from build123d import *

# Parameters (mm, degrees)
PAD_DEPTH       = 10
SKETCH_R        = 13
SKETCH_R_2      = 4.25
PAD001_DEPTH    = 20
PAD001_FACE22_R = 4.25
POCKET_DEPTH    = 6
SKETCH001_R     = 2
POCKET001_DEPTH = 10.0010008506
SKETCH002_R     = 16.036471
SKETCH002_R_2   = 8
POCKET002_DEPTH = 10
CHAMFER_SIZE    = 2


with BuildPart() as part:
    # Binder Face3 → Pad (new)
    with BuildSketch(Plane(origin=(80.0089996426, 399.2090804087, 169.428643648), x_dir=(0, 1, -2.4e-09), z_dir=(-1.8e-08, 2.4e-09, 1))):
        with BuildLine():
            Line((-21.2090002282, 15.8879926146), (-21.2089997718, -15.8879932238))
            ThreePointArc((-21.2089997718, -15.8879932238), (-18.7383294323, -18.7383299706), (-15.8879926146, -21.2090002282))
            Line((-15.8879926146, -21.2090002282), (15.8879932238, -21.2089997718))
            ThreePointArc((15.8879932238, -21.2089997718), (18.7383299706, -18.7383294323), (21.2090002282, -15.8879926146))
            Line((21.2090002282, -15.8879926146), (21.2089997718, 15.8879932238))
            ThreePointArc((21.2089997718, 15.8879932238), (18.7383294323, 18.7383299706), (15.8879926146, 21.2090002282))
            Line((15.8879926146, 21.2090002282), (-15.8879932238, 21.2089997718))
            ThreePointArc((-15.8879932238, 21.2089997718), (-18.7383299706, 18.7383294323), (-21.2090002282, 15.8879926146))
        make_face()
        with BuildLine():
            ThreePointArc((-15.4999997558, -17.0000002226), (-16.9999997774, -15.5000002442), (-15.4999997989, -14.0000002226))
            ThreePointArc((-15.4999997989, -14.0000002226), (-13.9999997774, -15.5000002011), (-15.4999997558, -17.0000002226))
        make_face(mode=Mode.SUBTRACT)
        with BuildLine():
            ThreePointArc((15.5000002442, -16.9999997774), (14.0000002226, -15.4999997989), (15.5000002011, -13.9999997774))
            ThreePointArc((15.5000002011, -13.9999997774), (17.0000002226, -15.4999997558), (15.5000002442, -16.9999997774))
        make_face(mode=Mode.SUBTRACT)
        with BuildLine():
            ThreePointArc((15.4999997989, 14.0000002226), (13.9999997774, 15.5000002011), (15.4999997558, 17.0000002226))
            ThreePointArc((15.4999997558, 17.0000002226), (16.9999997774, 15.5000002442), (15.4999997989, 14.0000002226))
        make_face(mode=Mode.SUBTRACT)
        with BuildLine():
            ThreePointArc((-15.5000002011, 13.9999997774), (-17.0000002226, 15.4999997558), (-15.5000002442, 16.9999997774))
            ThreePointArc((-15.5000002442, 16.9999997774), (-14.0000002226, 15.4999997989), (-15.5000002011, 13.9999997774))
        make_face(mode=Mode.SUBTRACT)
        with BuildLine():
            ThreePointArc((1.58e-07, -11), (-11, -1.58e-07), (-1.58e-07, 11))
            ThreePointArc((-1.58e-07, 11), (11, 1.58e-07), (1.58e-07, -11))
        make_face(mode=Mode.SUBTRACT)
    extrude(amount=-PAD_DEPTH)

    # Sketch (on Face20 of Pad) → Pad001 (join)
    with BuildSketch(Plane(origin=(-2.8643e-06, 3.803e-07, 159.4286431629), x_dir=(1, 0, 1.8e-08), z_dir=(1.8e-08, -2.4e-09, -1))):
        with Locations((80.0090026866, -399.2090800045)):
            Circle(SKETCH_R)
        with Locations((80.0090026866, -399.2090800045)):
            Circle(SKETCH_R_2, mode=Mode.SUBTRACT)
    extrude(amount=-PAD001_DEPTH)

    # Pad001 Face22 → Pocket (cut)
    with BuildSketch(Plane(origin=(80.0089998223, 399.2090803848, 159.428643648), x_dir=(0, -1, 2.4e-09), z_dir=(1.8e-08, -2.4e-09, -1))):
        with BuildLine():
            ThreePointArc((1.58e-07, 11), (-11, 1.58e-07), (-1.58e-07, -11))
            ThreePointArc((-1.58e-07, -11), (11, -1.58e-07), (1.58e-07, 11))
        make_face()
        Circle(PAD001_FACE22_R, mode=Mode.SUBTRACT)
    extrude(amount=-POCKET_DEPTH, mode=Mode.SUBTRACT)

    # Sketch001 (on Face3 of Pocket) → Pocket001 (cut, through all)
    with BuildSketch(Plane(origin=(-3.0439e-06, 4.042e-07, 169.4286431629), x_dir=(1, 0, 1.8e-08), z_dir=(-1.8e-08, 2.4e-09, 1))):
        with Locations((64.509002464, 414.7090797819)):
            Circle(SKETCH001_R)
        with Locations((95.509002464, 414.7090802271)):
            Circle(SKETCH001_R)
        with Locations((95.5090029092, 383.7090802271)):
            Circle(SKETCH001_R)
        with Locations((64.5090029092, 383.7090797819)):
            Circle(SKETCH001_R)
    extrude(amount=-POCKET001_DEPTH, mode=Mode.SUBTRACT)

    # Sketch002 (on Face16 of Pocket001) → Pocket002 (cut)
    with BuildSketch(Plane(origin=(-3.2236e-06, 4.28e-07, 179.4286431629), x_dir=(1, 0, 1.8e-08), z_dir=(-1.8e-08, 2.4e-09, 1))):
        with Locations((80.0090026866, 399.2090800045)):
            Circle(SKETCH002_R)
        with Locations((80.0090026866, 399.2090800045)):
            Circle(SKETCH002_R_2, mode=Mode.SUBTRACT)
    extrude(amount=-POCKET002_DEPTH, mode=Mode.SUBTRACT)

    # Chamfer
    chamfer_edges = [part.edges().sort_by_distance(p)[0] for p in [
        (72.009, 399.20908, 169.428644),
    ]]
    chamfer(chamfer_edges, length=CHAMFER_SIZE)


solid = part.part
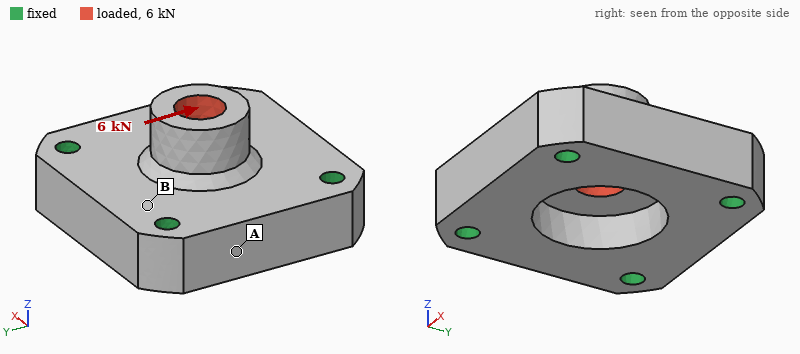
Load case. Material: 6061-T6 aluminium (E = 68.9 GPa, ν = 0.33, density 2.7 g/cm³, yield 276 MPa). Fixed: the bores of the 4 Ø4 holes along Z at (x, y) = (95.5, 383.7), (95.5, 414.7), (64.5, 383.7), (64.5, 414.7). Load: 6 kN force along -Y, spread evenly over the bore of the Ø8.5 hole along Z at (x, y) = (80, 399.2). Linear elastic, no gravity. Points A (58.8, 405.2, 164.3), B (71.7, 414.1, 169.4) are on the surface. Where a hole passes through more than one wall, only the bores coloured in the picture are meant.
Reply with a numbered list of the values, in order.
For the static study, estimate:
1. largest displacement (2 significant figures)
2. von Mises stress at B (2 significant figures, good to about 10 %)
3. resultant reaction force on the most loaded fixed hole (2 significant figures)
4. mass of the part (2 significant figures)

1. 25 µm
2. 15 MPa
3. 1.8 kN
4. 43 g
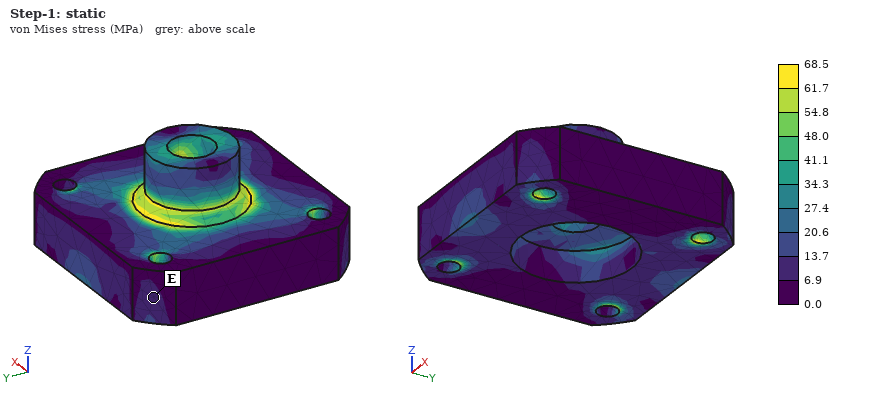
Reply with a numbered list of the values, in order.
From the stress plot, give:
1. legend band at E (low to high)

1. 6.9 to 13.7 MPa
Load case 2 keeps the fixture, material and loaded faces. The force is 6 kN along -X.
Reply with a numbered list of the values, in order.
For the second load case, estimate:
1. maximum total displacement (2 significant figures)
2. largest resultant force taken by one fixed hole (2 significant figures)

1. 25 µm
2. 1.8 kN
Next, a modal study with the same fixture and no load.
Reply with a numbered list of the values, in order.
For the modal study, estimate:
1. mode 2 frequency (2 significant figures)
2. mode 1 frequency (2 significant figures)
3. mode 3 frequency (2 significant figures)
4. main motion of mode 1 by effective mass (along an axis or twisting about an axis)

1. 32 kHz
2. 27 kHz
3. 32 kHz
4. along Z
